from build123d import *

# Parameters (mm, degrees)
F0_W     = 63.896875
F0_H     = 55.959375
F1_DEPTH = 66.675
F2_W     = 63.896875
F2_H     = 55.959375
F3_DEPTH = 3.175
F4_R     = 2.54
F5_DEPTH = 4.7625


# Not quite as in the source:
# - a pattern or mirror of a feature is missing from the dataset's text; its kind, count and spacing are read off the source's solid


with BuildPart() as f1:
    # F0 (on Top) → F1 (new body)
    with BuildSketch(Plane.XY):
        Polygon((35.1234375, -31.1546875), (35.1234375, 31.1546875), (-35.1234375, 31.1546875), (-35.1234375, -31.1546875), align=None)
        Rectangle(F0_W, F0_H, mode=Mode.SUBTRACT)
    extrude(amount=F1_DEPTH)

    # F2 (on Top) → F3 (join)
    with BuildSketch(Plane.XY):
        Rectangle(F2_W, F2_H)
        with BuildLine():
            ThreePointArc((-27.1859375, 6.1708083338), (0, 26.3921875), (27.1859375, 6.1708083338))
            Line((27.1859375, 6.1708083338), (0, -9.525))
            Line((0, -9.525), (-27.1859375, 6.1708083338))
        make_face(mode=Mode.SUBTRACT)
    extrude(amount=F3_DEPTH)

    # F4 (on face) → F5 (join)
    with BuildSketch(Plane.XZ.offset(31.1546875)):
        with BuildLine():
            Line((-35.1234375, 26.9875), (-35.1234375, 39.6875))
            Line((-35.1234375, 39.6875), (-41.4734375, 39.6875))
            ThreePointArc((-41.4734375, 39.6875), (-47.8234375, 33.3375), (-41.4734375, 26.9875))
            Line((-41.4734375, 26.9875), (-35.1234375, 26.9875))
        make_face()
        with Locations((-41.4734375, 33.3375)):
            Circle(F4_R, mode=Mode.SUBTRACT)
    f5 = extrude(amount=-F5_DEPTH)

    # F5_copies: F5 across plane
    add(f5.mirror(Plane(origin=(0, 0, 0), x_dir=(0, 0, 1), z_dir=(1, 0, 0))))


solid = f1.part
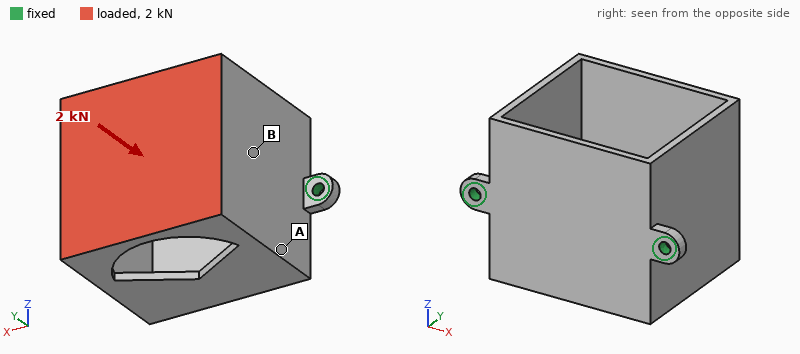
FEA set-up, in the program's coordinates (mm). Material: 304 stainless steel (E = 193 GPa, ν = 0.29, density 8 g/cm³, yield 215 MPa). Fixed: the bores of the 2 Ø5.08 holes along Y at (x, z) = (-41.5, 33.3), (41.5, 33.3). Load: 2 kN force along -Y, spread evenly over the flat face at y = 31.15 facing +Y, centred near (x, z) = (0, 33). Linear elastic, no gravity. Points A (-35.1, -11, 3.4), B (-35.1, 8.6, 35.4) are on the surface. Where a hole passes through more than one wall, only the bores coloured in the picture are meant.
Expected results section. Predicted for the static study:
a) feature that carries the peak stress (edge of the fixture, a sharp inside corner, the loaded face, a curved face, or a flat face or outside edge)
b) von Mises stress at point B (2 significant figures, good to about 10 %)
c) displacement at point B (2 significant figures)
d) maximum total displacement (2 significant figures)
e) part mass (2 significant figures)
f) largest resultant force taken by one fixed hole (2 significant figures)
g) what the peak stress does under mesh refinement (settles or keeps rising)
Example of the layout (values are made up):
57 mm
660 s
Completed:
edge of the fixture
12 MPa
17 µm
96 µm
500 g
1.0 kN
keeps rising
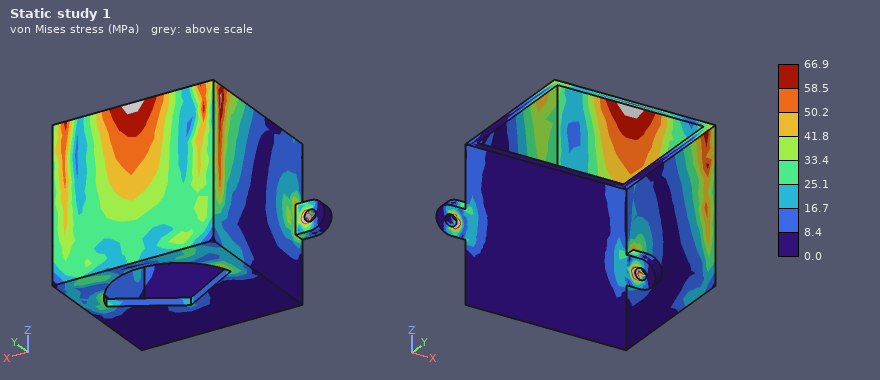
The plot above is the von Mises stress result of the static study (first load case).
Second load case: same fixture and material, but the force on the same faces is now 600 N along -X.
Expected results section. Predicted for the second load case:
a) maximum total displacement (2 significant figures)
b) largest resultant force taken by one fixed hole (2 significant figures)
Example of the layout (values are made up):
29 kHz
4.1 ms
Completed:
0.18 mm
550 N
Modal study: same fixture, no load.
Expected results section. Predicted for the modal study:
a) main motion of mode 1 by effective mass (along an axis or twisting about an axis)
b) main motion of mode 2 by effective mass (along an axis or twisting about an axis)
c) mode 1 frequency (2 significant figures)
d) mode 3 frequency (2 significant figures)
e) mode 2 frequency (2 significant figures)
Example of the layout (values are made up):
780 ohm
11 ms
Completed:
along Z
along X
540 Hz
2400 Hz
750 Hz
